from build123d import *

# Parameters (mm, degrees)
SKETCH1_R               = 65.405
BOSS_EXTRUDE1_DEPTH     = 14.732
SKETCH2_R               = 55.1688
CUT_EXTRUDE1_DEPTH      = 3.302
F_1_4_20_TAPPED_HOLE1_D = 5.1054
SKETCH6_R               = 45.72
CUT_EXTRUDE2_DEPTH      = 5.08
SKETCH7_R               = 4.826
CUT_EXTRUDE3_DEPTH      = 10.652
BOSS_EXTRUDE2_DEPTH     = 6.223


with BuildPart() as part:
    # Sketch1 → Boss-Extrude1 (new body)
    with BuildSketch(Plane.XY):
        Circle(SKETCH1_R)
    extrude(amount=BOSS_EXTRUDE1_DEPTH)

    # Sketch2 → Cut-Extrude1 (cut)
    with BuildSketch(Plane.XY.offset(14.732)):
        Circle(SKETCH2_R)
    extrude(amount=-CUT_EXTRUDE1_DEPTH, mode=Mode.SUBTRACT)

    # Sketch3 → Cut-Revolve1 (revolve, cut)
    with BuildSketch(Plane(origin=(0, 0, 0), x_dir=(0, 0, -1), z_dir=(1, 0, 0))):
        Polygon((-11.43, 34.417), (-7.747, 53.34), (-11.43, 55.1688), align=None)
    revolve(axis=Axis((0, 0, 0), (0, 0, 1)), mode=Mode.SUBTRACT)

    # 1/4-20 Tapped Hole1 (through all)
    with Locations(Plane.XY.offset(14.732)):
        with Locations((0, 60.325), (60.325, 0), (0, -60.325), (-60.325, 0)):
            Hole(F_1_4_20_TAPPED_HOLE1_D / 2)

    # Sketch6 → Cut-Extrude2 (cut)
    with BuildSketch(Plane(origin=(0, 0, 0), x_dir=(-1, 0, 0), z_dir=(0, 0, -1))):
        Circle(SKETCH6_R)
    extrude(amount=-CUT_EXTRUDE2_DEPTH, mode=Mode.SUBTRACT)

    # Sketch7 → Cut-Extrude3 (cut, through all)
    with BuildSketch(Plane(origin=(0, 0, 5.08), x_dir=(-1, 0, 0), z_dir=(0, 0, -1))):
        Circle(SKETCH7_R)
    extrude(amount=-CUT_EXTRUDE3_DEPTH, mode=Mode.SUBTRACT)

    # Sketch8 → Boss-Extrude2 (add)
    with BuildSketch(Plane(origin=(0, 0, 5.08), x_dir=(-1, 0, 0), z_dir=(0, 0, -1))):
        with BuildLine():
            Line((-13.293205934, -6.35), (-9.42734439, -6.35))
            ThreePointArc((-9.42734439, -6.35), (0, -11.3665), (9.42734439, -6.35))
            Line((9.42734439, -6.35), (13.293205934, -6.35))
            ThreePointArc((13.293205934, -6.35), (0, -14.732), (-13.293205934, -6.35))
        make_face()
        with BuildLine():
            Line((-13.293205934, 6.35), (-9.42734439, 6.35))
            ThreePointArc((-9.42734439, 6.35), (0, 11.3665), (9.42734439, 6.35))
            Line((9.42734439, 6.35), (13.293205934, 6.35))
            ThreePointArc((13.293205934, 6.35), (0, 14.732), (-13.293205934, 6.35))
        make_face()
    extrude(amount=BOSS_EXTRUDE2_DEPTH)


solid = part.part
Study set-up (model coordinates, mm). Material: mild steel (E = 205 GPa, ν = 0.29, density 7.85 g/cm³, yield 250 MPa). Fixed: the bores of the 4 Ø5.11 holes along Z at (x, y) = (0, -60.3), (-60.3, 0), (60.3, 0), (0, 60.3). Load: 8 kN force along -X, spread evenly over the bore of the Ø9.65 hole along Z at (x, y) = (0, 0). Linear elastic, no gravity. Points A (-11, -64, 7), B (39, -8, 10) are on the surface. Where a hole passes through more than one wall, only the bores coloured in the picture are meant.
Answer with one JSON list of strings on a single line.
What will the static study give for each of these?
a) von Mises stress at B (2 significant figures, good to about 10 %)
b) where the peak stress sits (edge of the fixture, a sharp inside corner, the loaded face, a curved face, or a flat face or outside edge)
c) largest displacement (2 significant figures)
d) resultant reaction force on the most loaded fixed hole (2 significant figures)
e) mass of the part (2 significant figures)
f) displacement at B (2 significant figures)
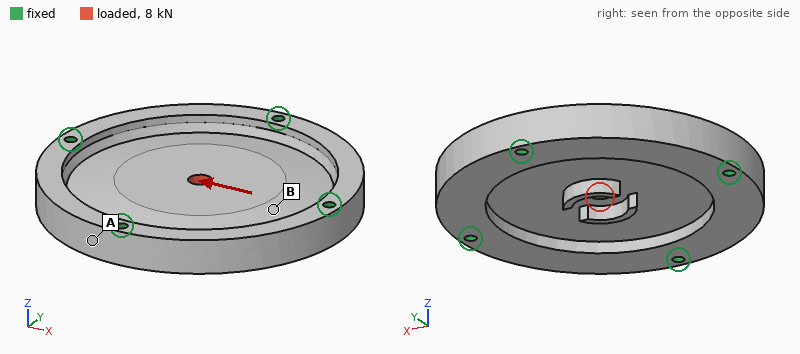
["13 MPa", "the loaded face", "5.9 µm", "2.2 kN", "950 g", "2.6 µm"]
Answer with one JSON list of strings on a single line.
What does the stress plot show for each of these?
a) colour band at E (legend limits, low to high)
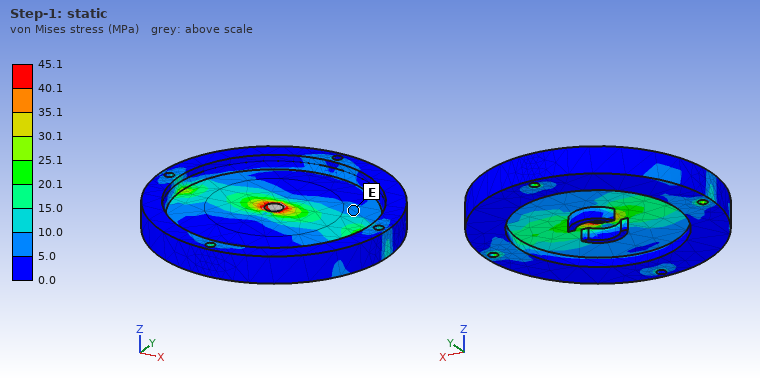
["5.0 to 10.0 MPa"]
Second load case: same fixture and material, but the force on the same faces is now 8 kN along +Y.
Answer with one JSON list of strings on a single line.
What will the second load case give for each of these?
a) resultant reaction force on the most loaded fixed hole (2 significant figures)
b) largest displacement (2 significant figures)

["2.2 kN", "5.9 µm"]
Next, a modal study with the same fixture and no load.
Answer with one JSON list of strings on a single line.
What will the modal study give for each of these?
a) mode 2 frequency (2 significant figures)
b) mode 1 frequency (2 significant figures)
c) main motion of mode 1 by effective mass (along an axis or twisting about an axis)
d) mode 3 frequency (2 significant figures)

["6700 Hz", "4300 Hz", "along Z", "6800 Hz"]
